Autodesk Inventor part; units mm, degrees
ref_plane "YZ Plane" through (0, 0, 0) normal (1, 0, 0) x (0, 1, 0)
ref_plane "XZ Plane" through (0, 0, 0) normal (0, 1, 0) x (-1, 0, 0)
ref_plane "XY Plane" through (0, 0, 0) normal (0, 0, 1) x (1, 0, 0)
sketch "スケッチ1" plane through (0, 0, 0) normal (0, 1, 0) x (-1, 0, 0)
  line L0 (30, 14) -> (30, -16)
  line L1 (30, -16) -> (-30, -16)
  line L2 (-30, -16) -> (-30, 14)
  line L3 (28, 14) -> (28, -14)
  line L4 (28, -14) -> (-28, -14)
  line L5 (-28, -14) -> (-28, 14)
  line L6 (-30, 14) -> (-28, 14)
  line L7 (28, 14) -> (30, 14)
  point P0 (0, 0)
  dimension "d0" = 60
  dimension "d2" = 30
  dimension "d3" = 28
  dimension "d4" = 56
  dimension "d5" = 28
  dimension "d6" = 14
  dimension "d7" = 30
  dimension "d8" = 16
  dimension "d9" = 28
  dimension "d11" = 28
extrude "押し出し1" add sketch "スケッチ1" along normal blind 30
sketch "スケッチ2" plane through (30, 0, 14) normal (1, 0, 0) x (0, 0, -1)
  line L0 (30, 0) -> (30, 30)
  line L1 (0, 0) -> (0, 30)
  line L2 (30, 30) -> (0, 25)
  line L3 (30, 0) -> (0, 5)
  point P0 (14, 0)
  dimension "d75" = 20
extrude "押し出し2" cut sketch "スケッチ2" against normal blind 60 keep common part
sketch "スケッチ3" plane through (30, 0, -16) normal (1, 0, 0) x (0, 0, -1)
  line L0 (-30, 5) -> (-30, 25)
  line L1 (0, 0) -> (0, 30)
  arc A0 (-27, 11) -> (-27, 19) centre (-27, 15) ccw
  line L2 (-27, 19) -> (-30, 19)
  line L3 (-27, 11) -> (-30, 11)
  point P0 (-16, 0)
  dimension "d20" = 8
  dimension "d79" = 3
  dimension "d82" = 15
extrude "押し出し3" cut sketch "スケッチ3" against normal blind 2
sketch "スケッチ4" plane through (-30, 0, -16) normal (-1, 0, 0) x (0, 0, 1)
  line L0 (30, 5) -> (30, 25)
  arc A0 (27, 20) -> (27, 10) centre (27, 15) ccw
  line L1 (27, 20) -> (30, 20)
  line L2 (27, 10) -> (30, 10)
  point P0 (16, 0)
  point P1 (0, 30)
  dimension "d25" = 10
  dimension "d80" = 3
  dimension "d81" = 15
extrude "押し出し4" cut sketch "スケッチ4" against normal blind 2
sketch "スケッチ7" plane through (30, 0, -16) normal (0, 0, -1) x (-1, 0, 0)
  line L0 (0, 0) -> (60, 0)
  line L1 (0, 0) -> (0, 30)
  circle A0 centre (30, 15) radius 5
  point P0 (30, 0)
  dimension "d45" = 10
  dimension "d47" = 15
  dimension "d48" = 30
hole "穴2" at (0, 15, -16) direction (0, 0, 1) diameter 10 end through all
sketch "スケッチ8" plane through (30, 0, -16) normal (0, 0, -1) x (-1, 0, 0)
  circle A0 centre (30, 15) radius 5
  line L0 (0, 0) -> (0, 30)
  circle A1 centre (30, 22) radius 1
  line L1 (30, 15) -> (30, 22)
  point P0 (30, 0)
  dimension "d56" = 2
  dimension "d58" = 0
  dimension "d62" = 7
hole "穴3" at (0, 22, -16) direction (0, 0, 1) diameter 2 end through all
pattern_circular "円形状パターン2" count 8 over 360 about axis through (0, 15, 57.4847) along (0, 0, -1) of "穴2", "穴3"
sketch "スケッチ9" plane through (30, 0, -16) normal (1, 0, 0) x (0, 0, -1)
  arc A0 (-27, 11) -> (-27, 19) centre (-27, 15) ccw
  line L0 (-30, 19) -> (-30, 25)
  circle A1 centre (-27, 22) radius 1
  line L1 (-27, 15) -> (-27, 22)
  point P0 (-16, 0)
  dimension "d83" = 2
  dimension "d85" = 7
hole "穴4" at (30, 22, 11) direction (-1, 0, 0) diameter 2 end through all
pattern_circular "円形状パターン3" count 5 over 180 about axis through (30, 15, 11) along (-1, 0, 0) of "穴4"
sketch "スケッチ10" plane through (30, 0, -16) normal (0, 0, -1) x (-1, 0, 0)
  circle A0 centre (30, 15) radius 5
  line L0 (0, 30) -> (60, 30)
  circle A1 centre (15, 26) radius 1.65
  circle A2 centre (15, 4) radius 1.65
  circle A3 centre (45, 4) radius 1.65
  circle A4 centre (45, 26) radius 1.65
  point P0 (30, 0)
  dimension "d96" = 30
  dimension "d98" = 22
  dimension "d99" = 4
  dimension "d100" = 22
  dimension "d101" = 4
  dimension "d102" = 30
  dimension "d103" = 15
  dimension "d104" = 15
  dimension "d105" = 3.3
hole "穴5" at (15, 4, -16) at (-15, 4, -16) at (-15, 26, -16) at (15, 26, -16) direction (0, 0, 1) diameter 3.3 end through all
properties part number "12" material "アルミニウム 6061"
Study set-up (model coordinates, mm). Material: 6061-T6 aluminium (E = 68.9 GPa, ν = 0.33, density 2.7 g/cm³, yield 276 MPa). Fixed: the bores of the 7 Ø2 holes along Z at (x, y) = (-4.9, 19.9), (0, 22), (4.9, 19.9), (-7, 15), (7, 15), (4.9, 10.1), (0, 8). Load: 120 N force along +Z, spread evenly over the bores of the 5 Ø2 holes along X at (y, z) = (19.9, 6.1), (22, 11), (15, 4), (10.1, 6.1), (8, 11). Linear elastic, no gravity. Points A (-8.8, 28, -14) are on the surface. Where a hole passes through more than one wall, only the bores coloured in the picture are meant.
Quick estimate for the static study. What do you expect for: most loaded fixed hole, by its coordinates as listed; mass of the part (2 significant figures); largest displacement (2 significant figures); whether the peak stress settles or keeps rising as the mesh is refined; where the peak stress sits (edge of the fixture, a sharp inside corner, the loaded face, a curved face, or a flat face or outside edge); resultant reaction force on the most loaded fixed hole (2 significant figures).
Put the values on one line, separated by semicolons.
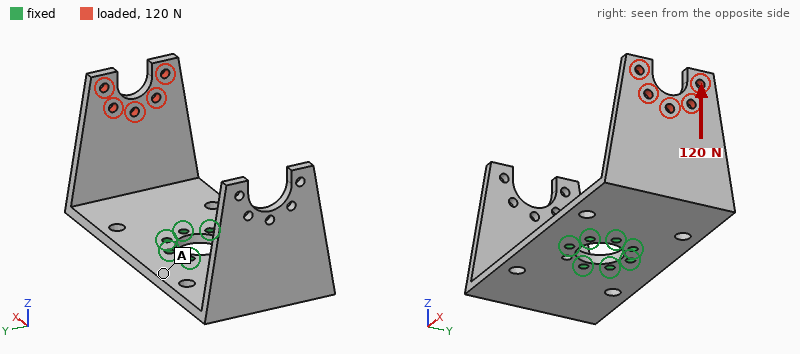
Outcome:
(7, 15); 16 g; 0.78 mm; keeps rising; edge of the fixture; 190 N
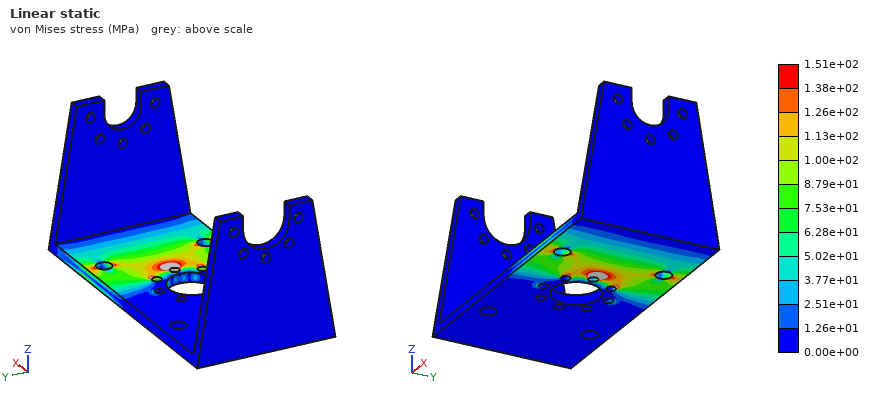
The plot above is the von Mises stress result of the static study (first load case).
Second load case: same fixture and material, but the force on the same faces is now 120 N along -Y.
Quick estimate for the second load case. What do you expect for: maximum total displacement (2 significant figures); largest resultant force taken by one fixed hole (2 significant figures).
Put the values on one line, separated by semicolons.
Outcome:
0.71 mm; 200 N
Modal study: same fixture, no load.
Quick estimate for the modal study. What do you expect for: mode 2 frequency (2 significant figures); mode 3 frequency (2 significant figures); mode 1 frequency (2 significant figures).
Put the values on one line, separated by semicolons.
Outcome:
1000 Hz; 1700 Hz; 990 Hz
